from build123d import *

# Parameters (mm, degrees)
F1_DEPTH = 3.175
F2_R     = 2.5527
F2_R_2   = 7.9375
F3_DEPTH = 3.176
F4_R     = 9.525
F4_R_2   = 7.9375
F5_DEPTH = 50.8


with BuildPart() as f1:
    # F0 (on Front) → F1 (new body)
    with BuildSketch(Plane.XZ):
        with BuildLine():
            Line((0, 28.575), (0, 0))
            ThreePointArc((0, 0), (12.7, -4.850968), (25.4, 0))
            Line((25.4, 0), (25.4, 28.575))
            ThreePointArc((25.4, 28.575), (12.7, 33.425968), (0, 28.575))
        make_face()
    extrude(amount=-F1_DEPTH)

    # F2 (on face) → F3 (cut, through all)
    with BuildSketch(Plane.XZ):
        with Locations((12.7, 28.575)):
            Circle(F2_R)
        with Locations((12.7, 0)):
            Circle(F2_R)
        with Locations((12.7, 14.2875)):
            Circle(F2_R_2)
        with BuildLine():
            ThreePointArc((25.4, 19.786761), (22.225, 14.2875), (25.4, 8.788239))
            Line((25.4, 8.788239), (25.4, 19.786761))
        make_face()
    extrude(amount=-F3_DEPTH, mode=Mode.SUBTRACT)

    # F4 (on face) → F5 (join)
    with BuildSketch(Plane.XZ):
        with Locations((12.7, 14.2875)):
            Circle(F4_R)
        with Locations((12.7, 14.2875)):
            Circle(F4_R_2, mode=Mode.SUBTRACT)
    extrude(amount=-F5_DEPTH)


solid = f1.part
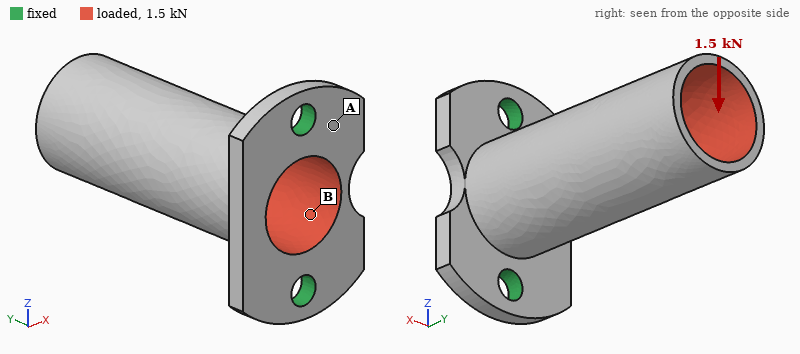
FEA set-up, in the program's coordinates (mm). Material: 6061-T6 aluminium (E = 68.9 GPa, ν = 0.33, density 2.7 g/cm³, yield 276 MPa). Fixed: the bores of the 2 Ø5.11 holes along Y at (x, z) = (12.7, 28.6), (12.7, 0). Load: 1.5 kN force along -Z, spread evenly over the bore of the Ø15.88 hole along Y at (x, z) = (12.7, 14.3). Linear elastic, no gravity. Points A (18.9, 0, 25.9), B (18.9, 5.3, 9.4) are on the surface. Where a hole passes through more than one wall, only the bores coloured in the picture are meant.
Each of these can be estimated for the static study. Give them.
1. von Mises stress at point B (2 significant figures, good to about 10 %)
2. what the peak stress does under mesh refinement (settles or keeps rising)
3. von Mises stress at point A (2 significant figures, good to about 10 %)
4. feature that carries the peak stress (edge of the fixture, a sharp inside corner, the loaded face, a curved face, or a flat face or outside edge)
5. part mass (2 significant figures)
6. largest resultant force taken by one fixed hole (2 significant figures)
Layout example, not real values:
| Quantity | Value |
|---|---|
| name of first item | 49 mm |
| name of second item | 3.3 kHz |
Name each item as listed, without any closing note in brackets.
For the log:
| Quantity | Value |
|---|---|
| von Mises stress at point B | 66 MPa |
| what the peak stress does under mesh refinement | keeps rising |
| von Mises stress at point A | 28 MPa |
| feature that carries the peak stress | edge of the fixture |
| part mass | 17 g |
| largest resultant force taken by one fixed hole | 1.9 kN |
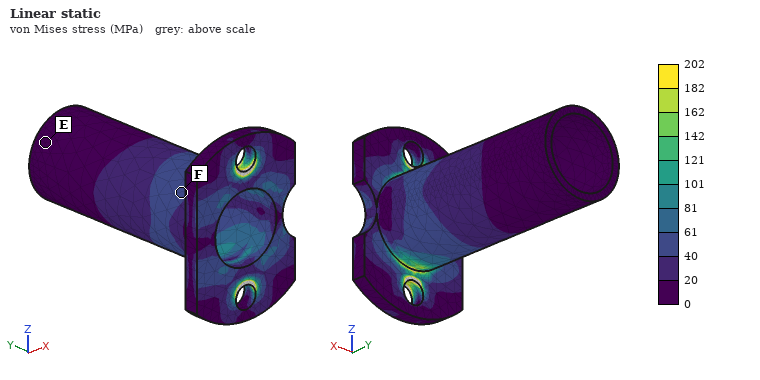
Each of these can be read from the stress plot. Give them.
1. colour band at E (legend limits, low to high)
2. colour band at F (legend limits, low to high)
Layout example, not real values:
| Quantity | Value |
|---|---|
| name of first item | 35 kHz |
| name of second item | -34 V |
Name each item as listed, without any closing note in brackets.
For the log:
| Quantity | Value |
|---|---|
| colour band at E | 0 to 20 MPa |
| colour band at F | 40 to 61 MPa |
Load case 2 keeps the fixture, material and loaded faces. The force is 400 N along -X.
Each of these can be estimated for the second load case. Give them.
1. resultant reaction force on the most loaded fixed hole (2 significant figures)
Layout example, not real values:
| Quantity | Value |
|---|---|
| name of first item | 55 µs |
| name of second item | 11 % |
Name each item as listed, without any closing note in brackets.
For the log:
| Quantity | Value |
|---|---|
| resultant reaction force on the most loaded fixed hole | 200 N |
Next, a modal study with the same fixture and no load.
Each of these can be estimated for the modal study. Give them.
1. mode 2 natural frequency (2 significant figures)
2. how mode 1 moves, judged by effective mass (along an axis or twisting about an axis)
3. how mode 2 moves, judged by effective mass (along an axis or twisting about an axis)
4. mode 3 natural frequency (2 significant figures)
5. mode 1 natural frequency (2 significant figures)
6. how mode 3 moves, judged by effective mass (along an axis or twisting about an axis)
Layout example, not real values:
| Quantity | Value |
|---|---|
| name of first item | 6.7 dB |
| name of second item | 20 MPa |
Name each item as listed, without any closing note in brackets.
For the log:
| Quantity | Value |
|---|---|
| mode 2 natural frequency | 4600 Hz |
| how mode 1 moves, judged by effective mass | along X |
| how mode 2 moves, judged by effective mass | along Z |
| mode 3 natural frequency | 13 kHz |
| mode 1 natural frequency | 2100 Hz |
| how mode 3 moves, judged by effective mass | along Y |
